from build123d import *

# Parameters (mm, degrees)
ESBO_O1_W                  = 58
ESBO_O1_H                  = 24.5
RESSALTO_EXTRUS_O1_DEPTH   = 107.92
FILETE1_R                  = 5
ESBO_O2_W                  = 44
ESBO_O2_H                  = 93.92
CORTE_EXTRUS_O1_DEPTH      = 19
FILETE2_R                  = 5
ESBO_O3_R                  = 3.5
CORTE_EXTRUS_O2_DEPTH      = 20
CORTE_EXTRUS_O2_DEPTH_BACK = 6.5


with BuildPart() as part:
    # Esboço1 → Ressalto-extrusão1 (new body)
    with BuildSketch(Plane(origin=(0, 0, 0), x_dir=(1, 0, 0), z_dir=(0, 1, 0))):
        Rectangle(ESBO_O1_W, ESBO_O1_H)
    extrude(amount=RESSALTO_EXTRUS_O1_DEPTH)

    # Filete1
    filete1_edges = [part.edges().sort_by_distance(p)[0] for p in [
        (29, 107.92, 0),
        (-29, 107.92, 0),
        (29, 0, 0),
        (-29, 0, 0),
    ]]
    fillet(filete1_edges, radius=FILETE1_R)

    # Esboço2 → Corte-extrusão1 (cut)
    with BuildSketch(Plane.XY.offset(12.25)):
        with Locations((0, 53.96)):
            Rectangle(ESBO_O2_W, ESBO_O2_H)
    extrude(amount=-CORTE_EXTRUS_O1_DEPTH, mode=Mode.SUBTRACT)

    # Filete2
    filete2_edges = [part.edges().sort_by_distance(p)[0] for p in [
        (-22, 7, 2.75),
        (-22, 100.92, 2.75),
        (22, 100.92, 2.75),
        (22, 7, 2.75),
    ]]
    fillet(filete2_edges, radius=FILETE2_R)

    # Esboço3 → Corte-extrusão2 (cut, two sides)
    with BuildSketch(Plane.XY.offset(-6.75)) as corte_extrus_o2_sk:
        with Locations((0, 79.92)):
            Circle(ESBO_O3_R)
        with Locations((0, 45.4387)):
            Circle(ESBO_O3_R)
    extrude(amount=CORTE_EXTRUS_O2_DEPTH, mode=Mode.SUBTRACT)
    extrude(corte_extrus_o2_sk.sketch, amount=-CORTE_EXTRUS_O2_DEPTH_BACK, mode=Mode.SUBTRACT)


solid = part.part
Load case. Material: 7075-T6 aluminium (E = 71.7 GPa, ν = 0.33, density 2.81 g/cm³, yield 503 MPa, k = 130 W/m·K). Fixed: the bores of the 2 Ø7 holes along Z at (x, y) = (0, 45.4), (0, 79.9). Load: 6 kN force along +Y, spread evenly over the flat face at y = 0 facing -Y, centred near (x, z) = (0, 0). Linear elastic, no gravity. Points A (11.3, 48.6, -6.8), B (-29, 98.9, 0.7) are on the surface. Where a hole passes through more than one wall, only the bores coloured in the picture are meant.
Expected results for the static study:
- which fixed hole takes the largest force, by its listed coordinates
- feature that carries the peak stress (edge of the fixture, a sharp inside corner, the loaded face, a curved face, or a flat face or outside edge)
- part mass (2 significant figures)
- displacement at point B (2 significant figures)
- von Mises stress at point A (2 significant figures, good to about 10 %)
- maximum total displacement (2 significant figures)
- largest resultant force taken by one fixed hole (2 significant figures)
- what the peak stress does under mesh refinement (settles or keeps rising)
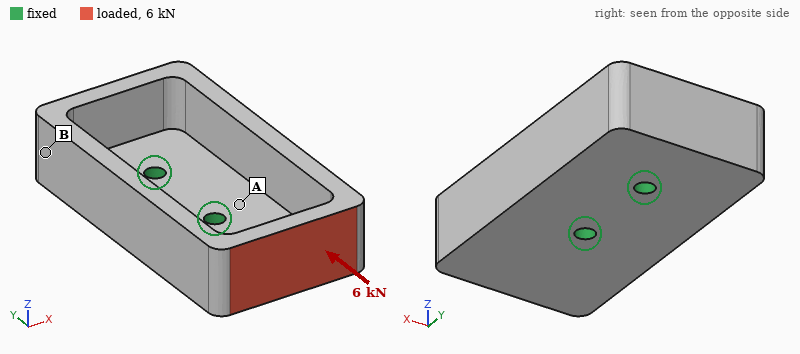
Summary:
(0, 45.4)
edge of the fixture
210 g
0.040 mm
27 MPa
0.14 mm
3.8 kN
keeps rising
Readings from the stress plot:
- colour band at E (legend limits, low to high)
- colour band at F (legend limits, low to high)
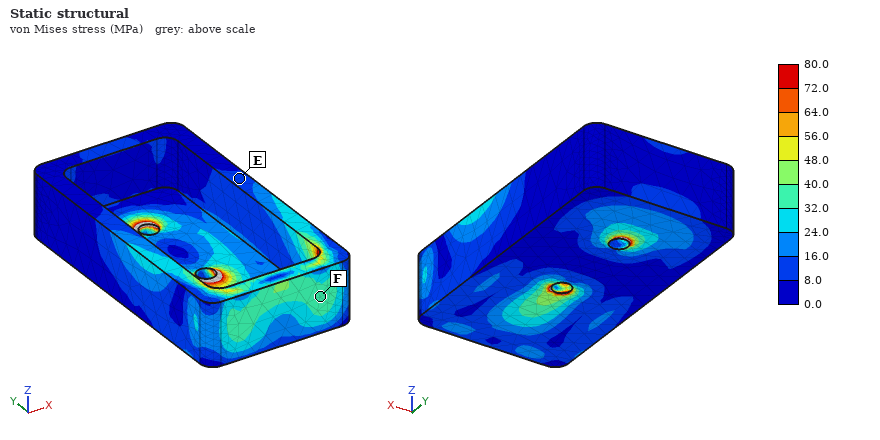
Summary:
8.0 to 16.0 MPa
32.0 to 40.0 MPa
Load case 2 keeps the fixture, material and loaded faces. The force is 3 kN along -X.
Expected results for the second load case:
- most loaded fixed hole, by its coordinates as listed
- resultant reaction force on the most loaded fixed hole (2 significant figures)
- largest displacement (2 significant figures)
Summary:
(0, 45.4)
6.2 kN
0.21 mm
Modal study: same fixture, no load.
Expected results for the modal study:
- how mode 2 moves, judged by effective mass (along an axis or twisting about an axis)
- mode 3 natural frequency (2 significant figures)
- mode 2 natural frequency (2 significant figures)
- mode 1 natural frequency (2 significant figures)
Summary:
along Z
2900 Hz
2000 Hz
1800 Hz
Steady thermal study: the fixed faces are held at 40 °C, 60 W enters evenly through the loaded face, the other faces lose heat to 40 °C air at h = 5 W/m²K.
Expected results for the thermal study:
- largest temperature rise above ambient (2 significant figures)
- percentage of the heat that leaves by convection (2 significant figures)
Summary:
54 K
3.7 %
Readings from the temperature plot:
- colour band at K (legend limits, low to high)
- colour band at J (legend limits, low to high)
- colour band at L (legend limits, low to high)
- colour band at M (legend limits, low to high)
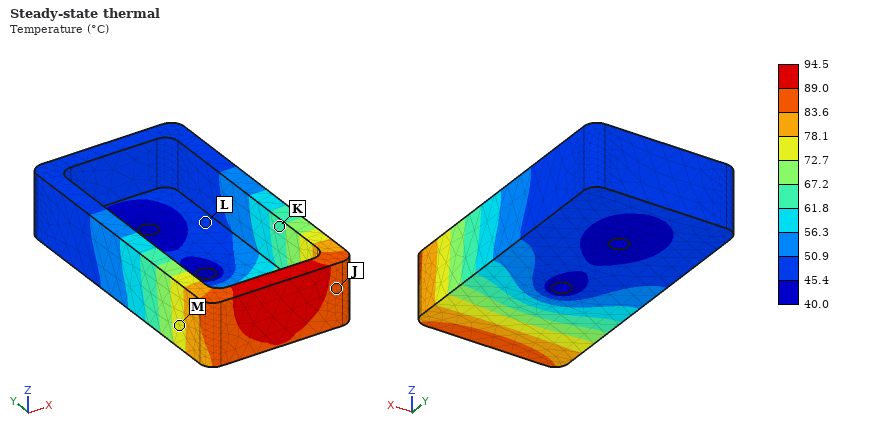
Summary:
61.8 to 67.2 °C
83.6 to 89.0 °C
45.4 to 50.9 °C
72.7 to 78.1 °C
